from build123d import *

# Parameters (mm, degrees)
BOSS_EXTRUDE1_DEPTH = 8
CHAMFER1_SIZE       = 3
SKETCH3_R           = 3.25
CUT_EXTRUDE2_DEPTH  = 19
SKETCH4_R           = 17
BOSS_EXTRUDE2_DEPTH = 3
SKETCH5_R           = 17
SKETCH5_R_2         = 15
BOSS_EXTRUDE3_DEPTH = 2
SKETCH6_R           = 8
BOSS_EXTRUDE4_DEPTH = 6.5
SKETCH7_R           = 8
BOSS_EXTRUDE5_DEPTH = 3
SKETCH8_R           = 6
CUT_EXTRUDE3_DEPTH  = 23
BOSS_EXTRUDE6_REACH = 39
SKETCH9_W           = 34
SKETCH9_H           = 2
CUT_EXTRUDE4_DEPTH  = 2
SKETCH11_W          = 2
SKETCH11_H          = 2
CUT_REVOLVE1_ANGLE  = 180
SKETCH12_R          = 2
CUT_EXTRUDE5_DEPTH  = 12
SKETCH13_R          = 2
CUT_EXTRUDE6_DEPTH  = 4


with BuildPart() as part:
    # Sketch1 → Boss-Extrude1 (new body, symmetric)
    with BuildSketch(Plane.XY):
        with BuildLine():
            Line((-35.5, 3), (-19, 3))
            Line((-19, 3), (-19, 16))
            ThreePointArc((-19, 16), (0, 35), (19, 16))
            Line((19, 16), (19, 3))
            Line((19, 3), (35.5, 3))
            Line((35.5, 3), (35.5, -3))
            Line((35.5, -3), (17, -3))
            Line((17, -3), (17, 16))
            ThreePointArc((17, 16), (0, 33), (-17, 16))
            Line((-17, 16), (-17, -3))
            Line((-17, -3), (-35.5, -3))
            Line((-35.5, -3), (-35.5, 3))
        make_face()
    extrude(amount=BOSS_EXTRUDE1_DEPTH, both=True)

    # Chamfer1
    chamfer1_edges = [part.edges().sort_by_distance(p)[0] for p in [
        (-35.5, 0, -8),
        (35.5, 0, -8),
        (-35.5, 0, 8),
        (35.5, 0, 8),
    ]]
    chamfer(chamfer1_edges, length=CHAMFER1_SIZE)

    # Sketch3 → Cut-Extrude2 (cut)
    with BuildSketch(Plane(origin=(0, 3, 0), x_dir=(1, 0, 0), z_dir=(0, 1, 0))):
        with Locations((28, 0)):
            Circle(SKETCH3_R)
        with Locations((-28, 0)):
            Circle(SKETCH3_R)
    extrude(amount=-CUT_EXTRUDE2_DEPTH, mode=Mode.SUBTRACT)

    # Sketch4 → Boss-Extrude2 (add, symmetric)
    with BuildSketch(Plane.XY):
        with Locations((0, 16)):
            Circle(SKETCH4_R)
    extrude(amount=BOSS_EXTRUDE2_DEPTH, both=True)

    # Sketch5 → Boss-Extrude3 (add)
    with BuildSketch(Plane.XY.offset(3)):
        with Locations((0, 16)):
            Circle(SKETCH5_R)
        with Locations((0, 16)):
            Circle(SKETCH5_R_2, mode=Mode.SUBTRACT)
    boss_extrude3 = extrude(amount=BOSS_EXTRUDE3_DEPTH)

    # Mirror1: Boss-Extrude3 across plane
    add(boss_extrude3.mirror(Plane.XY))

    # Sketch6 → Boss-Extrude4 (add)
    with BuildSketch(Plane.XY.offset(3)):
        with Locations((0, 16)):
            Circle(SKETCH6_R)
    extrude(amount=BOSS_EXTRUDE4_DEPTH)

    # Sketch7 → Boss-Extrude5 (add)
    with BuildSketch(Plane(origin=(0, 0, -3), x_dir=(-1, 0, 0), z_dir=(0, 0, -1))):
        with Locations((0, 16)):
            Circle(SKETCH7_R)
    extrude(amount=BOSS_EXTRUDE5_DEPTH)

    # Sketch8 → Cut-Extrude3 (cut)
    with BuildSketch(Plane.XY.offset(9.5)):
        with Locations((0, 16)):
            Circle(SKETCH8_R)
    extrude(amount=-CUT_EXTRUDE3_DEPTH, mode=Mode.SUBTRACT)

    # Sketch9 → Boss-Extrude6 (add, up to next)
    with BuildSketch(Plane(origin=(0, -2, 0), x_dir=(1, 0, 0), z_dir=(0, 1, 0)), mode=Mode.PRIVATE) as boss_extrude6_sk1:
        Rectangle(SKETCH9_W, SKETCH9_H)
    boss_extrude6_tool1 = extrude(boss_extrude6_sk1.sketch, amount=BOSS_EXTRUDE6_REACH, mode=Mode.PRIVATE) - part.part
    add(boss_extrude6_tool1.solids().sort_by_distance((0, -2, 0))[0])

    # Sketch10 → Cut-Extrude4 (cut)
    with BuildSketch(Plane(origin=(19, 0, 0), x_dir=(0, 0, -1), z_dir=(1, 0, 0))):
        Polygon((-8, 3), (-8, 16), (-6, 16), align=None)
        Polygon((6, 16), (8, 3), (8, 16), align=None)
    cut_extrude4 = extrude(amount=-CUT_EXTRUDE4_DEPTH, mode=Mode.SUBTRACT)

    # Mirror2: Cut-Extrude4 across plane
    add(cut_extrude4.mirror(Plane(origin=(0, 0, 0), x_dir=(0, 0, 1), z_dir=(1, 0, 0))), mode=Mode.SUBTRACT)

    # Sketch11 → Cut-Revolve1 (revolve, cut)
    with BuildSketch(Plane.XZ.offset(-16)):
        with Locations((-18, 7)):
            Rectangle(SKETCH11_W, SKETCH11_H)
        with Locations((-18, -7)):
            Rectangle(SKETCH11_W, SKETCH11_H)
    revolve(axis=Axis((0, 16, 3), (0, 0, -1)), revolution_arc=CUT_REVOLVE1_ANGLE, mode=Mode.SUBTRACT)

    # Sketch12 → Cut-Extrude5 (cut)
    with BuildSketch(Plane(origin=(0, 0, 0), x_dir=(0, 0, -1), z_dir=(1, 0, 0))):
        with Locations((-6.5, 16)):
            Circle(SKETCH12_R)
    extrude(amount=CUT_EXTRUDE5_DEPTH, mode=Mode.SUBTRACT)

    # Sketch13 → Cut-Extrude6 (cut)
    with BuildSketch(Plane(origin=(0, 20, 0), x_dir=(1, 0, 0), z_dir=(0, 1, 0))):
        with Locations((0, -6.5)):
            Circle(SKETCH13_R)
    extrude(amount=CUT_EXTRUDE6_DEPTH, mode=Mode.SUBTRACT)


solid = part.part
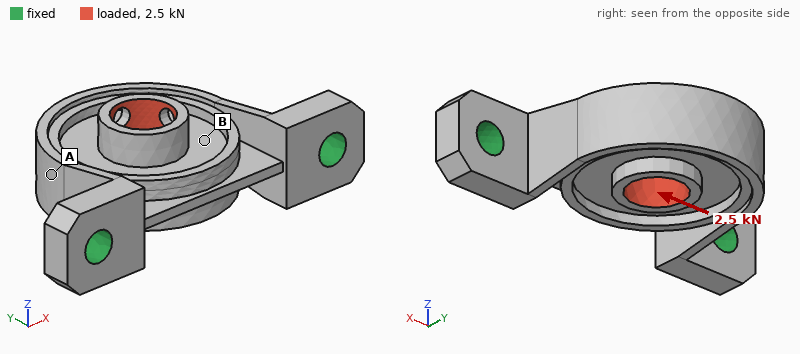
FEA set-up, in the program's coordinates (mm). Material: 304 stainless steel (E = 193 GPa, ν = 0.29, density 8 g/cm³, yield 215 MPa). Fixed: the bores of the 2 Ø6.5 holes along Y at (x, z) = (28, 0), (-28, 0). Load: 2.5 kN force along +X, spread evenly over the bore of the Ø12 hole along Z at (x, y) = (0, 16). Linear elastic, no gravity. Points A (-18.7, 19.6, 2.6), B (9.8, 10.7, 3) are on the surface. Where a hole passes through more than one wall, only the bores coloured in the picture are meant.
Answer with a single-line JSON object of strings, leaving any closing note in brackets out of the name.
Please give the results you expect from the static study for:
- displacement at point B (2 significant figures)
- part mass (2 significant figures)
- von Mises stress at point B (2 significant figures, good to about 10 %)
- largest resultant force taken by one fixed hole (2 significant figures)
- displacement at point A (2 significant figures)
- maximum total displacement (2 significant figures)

{"displacement at point B": "6.7 µm", "part mass": "94 g", "von Mises stress at point B": "22 MPa", "largest resultant force taken by one fixed hole": "1.6 kN", "displacement at point A": "10 µm", "maximum total displacement": "14 µm"}
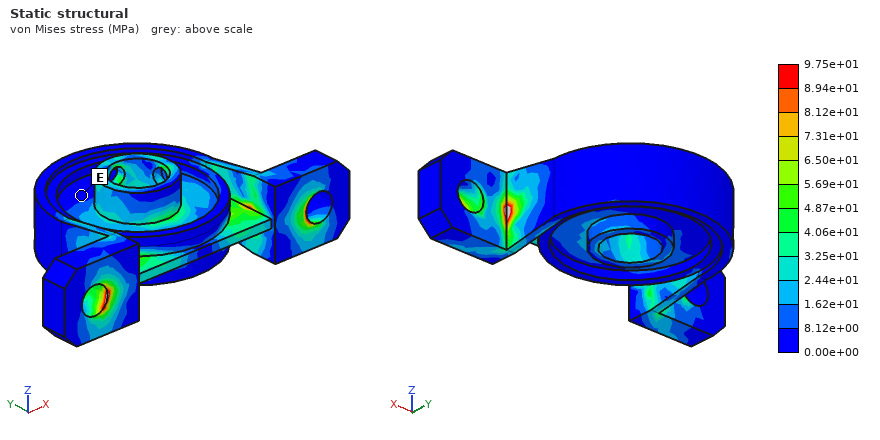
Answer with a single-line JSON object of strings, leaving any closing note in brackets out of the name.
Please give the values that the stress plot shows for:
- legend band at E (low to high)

{"legend band at E": "0.00e+00 to 8.12e+00 MPa"}
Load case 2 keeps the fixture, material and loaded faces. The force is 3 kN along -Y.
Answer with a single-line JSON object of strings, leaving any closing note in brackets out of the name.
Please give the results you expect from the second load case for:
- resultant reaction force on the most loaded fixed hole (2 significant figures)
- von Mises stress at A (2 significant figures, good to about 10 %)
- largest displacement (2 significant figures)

{"resultant reaction force on the most loaded fixed hole": "1.6 kN", "von Mises stress at A": "18 MPa", "largest displacement": "23 µm"}
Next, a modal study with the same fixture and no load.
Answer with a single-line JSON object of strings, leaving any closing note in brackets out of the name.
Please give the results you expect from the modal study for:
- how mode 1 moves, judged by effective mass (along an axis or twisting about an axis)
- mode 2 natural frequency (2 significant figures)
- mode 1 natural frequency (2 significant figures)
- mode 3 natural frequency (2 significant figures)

{"how mode 1 moves, judged by effective mass": "along Z", "mode 2 natural frequency": "9000 Hz", "mode 1 natural frequency": "3100 Hz", "mode 3 natural frequency": "9300 Hz"}
